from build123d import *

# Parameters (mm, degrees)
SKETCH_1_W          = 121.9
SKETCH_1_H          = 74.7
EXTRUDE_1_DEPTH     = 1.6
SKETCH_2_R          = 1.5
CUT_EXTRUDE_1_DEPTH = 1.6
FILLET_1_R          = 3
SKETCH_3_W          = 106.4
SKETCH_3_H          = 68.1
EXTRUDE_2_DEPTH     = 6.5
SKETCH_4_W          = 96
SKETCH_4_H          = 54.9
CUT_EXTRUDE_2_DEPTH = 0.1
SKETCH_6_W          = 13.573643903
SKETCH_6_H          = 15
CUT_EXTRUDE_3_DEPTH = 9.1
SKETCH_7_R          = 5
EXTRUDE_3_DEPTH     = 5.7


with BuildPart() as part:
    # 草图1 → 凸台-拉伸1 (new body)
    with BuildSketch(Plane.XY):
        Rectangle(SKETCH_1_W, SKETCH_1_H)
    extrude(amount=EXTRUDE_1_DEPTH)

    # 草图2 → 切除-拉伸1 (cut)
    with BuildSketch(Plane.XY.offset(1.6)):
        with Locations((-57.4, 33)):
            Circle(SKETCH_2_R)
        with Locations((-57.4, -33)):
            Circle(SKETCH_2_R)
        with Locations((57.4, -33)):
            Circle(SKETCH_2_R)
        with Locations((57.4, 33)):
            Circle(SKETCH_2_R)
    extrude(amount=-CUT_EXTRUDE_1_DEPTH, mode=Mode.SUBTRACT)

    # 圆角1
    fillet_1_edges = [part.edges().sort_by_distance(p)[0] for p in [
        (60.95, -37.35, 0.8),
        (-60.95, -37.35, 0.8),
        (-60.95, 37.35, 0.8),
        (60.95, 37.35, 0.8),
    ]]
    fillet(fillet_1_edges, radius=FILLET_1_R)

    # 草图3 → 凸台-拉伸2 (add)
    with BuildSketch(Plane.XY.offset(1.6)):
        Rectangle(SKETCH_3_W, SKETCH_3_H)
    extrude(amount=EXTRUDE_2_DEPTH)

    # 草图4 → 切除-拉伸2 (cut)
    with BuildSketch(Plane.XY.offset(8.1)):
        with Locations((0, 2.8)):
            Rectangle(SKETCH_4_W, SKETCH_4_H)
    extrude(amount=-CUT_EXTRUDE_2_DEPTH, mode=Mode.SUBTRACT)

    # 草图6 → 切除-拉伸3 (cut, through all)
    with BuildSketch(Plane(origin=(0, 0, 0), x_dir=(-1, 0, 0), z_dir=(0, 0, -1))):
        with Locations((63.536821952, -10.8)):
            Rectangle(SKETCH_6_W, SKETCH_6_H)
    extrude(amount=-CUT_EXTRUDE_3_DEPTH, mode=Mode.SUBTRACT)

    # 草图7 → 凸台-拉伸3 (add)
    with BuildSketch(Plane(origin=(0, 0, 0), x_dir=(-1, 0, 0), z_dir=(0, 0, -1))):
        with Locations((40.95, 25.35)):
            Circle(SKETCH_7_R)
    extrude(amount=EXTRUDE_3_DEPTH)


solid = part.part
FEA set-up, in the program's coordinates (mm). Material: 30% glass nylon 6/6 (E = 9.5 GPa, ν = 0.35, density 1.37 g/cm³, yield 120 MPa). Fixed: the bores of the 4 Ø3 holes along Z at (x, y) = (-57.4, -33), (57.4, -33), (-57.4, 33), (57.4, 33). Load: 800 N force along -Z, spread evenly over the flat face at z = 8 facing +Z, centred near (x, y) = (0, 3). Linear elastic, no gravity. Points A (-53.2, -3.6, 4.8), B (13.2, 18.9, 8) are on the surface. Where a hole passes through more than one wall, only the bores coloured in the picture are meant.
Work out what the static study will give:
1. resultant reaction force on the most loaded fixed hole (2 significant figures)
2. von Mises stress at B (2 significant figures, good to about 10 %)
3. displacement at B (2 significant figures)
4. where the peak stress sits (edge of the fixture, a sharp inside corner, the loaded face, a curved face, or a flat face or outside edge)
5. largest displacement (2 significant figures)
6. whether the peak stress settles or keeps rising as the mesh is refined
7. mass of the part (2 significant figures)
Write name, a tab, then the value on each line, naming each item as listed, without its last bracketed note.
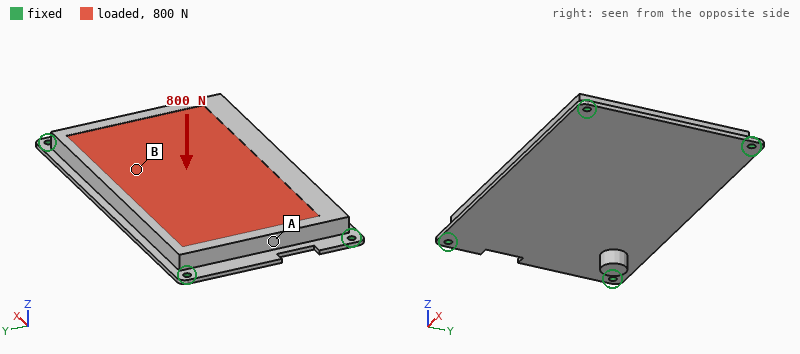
resultant reaction force on the most loaded fixed hole	530 N
von Mises stress at B	13 MPa
displacement at B	0.44 mm
where the peak stress sits	edge of the fixture
largest displacement	0.50 mm
whether the peak stress settles or keeps rising as the mesh is refined	keeps rising
mass of the part	84 g
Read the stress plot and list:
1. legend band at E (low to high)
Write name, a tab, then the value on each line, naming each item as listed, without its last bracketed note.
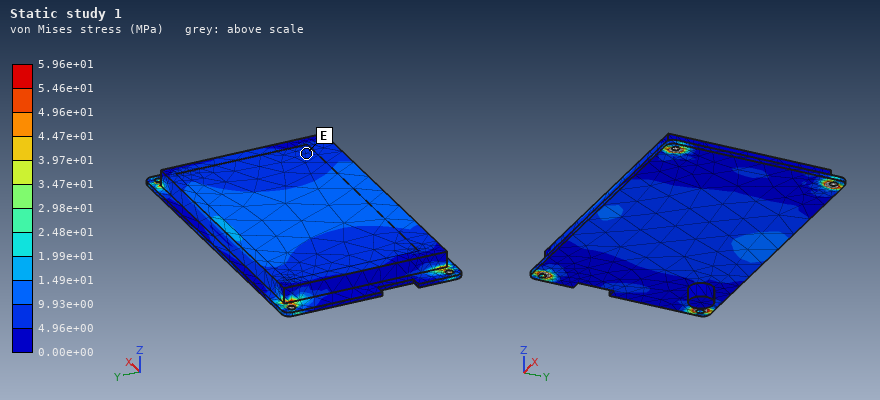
legend band at E	4.96e+00 to 9.93e+00 MPa
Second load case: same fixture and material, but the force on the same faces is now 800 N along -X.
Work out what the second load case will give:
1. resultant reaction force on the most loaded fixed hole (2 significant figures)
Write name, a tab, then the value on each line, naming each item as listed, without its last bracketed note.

resultant reaction force on the most loaded fixed hole	220 N
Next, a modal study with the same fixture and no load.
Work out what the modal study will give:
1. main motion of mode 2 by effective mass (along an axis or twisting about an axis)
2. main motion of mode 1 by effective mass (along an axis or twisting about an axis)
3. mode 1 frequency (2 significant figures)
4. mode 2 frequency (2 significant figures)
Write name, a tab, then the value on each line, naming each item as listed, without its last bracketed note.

main motion of mode 2 by effective mass	twisting about X
main motion of mode 1 by effective mass	along Z
mode 1 frequency	850 Hz
mode 2 frequency	1600 Hz
